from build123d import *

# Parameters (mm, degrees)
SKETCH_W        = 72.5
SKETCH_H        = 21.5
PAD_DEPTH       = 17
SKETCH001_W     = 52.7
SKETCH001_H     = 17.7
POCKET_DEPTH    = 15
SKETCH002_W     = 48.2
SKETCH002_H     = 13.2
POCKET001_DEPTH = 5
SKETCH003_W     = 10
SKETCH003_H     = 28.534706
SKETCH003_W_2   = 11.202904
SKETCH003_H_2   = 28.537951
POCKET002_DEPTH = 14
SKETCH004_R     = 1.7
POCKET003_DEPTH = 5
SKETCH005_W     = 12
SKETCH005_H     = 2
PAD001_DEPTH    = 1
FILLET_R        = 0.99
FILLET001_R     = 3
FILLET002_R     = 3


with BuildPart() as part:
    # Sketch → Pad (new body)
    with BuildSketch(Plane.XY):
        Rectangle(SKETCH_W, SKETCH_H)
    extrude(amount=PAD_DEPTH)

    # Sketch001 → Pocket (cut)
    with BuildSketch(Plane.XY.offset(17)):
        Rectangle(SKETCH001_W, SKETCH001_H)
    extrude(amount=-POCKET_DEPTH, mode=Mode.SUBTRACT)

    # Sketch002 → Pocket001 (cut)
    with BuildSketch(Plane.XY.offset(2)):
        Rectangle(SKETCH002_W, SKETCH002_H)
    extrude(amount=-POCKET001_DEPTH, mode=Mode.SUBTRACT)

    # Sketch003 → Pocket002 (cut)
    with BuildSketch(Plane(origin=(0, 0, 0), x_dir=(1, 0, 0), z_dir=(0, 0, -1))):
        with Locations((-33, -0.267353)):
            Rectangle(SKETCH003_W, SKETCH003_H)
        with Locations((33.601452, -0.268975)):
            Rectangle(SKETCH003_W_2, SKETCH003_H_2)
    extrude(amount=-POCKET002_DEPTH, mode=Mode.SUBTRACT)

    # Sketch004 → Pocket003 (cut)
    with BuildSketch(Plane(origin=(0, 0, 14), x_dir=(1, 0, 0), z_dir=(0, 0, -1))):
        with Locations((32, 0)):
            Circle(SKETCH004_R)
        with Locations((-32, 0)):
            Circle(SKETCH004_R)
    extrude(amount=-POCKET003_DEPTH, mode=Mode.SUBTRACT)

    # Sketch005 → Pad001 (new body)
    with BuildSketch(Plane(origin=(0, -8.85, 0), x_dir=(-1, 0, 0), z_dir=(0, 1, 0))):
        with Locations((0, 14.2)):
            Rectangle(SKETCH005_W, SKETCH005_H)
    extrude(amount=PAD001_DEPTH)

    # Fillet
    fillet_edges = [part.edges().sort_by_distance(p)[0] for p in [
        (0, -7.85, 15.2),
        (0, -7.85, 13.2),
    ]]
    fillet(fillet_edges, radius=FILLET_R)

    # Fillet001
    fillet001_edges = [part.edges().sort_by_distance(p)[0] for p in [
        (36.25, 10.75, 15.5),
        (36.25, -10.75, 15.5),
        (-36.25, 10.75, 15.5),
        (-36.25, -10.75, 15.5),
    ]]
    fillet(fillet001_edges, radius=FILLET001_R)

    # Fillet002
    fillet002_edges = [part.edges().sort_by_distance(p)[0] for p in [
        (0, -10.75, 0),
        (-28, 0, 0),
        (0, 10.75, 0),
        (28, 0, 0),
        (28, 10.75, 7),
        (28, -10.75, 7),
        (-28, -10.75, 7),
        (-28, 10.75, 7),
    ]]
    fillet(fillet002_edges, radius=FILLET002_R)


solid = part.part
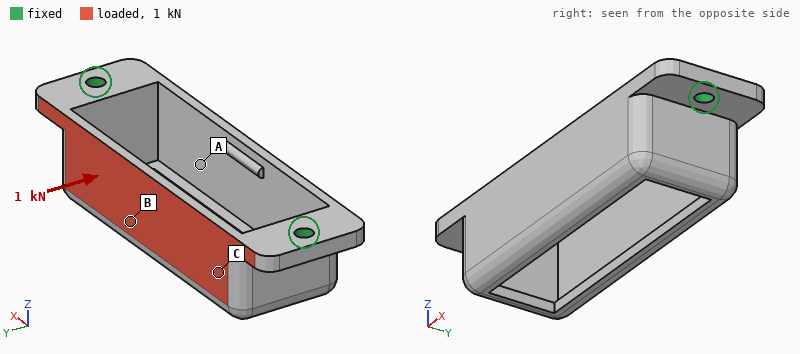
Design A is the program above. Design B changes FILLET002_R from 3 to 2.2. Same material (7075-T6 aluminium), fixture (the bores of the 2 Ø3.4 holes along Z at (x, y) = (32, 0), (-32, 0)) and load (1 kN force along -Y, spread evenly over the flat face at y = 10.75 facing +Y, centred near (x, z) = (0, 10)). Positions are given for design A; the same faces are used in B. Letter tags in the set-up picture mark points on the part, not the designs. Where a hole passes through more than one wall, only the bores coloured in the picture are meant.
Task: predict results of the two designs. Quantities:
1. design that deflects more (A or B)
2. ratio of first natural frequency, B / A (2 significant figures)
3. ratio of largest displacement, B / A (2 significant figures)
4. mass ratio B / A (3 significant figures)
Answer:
A
1.0
0.91
1.03
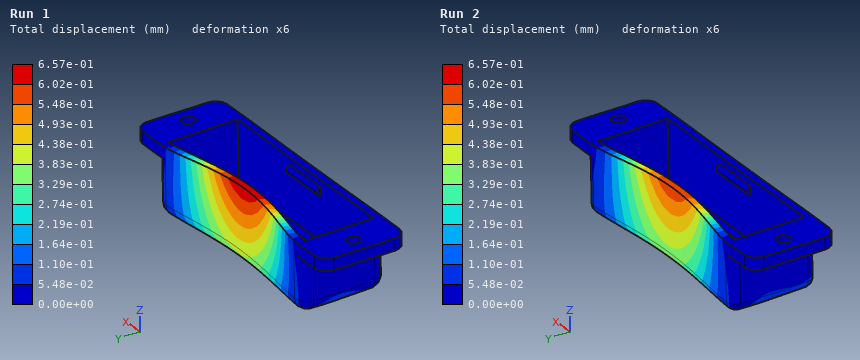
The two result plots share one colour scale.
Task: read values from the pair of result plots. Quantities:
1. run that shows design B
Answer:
Run 2
